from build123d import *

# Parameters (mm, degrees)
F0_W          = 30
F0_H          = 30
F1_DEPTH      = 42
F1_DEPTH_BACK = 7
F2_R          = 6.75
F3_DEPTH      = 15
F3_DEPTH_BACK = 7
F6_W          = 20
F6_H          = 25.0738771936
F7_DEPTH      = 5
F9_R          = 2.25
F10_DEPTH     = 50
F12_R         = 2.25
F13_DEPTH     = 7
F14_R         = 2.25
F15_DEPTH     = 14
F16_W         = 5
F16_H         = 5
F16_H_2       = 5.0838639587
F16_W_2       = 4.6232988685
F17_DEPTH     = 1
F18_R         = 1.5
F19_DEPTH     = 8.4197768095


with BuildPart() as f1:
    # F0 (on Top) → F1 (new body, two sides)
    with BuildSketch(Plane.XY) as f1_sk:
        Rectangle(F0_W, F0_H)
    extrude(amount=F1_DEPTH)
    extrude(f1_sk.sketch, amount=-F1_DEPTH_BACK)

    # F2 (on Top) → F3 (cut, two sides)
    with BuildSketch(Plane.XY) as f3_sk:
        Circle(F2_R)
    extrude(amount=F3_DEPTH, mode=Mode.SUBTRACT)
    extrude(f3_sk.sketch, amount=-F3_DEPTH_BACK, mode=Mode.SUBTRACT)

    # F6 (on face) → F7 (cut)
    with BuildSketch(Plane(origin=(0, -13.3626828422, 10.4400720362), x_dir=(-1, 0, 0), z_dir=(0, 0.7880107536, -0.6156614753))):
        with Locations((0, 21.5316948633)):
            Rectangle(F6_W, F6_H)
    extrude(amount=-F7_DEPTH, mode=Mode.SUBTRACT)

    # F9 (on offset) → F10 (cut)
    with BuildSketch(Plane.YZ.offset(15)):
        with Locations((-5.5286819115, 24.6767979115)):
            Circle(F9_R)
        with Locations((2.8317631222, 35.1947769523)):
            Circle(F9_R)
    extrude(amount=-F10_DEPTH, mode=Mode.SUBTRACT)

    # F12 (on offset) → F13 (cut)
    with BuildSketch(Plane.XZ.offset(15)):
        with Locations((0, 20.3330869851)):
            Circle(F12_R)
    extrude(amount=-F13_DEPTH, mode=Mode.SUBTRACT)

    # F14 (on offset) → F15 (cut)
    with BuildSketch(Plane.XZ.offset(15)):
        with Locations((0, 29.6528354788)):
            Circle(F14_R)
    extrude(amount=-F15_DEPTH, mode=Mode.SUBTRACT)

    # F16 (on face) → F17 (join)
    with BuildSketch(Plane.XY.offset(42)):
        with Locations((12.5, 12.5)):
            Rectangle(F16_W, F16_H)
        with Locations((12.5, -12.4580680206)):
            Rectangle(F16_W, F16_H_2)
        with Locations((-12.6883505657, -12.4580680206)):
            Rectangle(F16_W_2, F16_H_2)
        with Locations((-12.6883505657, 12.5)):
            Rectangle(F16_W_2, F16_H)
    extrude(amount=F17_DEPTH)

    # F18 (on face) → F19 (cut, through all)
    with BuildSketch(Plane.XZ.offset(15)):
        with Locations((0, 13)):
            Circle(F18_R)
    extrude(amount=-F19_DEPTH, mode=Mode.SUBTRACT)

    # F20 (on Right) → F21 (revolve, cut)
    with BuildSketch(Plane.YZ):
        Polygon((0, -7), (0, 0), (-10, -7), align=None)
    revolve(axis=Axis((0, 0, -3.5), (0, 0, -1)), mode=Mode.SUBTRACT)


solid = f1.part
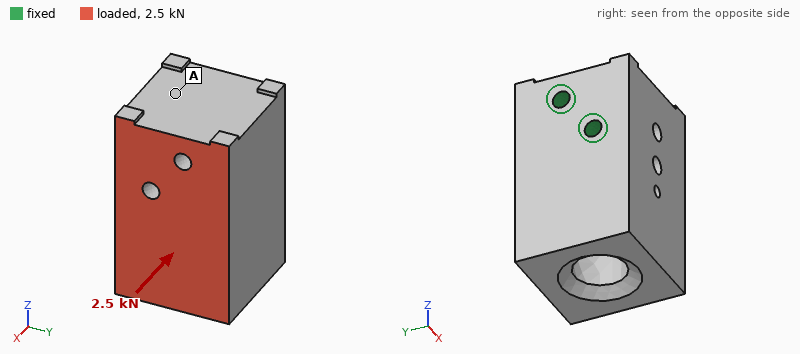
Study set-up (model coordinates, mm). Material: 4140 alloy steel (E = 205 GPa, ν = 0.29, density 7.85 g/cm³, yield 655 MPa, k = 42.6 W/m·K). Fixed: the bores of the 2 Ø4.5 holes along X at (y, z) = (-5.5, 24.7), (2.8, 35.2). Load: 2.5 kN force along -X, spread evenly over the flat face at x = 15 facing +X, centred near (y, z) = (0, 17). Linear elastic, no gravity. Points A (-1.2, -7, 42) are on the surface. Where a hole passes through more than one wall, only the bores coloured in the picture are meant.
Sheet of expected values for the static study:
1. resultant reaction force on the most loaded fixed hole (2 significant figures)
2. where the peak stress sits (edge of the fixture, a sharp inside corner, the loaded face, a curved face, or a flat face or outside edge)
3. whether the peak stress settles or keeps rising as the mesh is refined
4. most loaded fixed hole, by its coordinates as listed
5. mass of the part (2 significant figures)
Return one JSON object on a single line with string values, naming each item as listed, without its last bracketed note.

{"resultant reaction force on the most loaded fixed hole": "2.5 kN", "where the peak stress sits": "edge of the fixture", "whether the peak stress settles or keeps rising as the mesh is refined": "keeps rising", "most loaded fixed hole, by its coordinates as listed": "(-5.5, 24.7)", "mass of the part": "300 g"}
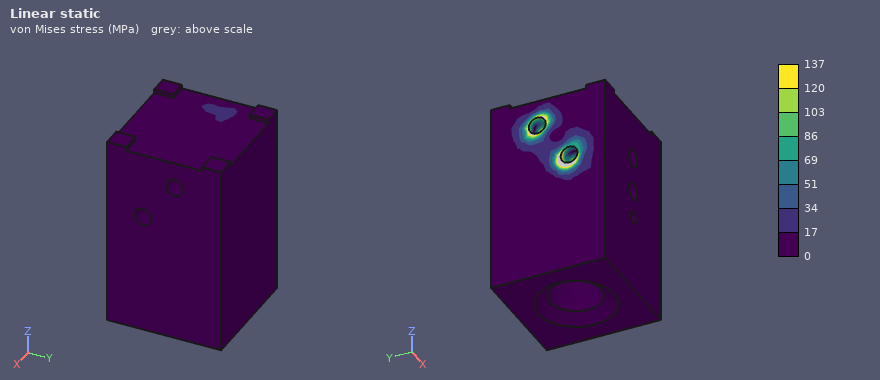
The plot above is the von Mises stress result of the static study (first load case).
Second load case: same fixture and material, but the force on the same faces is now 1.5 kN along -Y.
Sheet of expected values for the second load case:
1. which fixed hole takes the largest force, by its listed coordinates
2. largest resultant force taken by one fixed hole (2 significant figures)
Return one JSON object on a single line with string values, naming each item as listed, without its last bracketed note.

{"which fixed hole takes the largest force, by its listed coordinates": "(-5.5, 24.7)", "largest resultant force taken by one fixed hole": "2.3 kN"}
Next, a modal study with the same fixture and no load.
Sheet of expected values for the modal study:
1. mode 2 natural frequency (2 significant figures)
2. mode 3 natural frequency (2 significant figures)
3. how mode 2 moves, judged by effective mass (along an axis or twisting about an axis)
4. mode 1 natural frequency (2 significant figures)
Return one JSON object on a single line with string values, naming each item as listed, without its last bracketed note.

{"mode 2 natural frequency": "5200 Hz", "mode 3 natural frequency": "7700 Hz", "how mode 2 moves, judged by effective mass": "along Y", "mode 1 natural frequency": "2700 Hz"}
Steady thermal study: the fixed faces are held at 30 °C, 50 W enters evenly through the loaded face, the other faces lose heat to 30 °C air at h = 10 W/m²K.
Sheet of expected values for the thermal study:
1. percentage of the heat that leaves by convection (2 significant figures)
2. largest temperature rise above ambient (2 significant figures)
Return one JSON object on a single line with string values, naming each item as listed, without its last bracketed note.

{"percentage of the heat that leaves by convection": "6.7 %", "largest temperature rise above ambient": "62 K"}
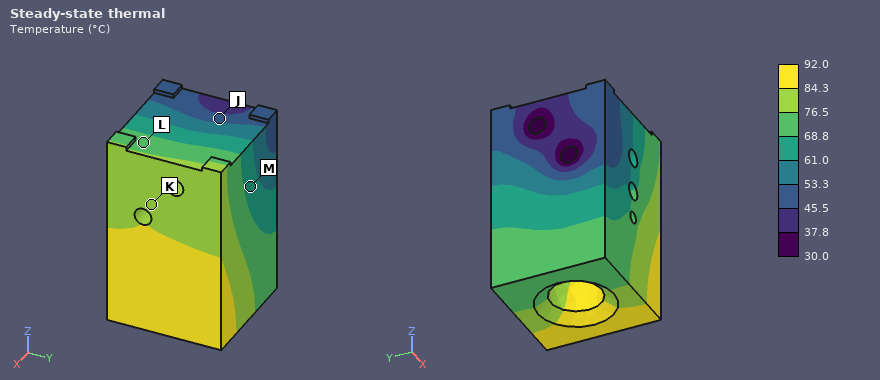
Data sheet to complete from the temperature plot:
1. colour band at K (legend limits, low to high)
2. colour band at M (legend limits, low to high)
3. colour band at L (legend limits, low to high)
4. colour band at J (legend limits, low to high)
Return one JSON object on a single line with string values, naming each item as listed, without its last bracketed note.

{"colour band at K": "76.5 to 84.3 °C", "colour band at M": "61.0 to 68.8 °C", "colour band at L": "68.8 to 76.5 °C", "colour band at J": "45.5 to 53.3 °C"}
